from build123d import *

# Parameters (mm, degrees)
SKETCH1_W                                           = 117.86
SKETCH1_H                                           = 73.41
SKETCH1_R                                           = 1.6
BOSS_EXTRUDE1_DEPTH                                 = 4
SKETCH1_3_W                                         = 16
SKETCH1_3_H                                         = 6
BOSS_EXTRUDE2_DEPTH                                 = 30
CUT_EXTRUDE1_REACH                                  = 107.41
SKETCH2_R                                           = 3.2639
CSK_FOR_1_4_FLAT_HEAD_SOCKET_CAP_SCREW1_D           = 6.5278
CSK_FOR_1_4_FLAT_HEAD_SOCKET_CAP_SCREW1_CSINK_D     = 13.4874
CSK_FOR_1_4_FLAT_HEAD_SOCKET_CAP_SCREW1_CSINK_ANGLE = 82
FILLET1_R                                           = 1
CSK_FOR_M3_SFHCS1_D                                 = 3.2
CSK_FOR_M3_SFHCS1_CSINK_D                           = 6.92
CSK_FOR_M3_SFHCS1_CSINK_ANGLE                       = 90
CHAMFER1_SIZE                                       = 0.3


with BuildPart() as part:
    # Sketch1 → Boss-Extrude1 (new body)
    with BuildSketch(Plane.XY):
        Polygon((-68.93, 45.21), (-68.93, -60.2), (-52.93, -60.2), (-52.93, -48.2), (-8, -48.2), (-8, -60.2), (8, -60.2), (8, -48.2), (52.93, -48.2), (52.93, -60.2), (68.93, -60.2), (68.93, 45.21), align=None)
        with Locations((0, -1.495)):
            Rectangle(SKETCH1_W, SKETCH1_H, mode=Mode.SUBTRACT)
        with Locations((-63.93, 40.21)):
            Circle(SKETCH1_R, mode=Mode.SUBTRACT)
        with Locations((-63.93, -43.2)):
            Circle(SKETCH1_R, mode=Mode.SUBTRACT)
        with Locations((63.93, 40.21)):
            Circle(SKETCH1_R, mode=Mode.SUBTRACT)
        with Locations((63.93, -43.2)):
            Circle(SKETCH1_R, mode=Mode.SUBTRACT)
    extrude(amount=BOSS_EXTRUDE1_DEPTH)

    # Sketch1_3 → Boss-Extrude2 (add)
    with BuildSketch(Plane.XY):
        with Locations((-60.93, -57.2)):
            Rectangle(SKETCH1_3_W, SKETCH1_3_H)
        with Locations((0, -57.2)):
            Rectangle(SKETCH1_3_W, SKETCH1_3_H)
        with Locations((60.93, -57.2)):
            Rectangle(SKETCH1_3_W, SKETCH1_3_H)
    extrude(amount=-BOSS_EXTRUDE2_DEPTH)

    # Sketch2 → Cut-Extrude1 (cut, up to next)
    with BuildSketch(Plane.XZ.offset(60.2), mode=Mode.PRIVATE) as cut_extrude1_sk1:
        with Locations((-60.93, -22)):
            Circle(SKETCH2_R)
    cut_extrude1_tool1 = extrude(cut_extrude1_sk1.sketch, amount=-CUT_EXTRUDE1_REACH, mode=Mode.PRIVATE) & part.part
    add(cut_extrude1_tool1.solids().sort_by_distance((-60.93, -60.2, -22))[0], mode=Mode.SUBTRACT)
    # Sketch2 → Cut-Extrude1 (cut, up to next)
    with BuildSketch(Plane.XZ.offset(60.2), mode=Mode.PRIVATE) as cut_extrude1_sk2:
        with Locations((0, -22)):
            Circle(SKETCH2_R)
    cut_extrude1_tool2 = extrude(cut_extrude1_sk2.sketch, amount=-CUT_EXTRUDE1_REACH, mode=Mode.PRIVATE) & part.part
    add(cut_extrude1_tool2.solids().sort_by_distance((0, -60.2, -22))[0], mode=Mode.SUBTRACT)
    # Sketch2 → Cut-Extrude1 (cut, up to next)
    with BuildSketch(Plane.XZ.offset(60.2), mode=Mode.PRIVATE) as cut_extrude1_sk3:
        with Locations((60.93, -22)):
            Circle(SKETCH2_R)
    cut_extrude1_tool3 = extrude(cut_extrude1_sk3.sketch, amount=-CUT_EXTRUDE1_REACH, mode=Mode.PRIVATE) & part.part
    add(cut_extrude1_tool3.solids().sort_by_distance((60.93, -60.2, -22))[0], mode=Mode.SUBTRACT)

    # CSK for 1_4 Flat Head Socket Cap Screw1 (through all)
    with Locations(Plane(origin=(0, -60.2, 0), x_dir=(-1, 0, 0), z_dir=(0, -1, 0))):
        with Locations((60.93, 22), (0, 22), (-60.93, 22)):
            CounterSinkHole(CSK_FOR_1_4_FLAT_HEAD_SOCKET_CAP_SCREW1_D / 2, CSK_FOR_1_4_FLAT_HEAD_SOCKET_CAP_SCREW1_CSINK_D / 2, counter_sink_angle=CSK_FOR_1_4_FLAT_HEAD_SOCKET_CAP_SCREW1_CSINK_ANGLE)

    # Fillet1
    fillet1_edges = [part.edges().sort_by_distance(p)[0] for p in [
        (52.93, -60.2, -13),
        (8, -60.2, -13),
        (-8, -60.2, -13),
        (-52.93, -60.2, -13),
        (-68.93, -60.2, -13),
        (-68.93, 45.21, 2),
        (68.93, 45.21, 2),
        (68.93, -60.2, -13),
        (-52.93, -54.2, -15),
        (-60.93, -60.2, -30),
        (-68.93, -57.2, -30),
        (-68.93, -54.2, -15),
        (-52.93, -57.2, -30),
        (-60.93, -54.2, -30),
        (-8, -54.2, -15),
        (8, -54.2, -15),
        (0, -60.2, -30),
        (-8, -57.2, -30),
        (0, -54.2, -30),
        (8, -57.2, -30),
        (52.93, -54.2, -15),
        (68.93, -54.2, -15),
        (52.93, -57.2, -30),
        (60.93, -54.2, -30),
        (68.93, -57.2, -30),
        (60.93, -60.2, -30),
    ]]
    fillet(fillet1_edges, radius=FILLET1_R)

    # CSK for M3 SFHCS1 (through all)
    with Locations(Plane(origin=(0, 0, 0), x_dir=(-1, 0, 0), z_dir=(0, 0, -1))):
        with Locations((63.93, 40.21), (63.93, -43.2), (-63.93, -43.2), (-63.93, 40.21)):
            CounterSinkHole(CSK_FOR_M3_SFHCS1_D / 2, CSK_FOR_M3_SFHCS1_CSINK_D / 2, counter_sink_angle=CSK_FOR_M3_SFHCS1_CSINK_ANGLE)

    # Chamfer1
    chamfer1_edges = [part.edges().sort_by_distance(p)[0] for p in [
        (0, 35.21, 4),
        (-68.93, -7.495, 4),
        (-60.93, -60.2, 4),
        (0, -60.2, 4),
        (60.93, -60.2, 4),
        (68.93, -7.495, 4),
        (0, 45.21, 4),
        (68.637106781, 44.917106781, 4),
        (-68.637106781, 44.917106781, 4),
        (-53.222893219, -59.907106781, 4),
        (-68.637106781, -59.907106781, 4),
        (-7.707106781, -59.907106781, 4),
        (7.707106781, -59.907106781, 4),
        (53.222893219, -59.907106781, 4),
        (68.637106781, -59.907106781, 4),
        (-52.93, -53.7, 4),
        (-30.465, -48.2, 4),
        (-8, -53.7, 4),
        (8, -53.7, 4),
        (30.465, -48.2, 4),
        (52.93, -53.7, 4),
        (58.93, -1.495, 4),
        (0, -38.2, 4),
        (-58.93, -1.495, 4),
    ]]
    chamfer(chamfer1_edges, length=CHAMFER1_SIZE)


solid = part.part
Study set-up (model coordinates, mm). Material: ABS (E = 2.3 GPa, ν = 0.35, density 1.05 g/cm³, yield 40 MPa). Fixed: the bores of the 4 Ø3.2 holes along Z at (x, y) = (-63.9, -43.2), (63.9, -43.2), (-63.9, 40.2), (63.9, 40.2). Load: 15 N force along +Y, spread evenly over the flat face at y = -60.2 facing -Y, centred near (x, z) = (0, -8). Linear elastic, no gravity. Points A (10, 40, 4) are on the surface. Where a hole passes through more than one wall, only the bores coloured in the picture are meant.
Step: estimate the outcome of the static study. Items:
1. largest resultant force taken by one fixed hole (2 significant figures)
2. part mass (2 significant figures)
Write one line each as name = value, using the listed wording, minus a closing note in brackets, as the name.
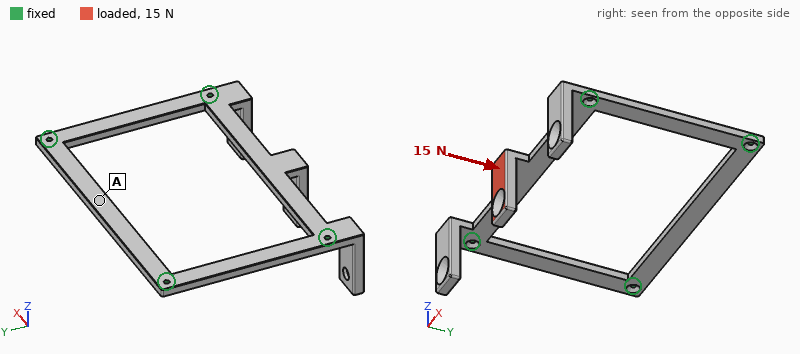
largest resultant force taken by one fixed hole = 5.2 N
part mass = 28 g
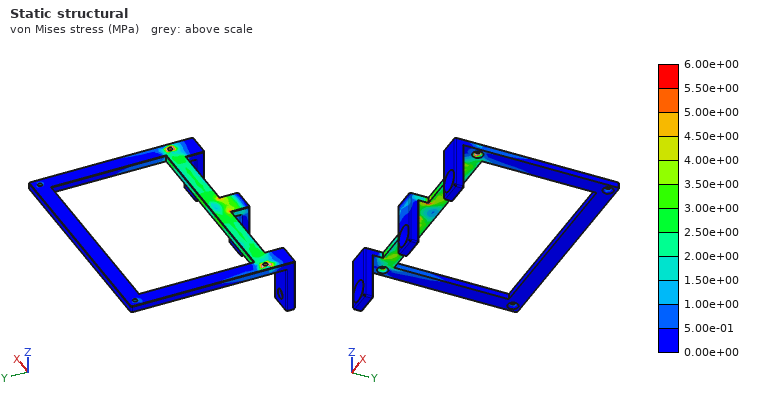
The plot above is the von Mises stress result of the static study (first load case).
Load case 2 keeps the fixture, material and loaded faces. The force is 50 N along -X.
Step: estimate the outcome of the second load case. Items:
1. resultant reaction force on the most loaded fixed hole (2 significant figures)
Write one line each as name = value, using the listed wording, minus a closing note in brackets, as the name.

resultant reaction force on the most loaded fixed hole = 26 N
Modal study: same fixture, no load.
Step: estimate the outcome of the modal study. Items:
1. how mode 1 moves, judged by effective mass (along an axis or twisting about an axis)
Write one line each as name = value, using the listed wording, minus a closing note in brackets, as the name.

how mode 1 moves, judged by effective mass = along Z
